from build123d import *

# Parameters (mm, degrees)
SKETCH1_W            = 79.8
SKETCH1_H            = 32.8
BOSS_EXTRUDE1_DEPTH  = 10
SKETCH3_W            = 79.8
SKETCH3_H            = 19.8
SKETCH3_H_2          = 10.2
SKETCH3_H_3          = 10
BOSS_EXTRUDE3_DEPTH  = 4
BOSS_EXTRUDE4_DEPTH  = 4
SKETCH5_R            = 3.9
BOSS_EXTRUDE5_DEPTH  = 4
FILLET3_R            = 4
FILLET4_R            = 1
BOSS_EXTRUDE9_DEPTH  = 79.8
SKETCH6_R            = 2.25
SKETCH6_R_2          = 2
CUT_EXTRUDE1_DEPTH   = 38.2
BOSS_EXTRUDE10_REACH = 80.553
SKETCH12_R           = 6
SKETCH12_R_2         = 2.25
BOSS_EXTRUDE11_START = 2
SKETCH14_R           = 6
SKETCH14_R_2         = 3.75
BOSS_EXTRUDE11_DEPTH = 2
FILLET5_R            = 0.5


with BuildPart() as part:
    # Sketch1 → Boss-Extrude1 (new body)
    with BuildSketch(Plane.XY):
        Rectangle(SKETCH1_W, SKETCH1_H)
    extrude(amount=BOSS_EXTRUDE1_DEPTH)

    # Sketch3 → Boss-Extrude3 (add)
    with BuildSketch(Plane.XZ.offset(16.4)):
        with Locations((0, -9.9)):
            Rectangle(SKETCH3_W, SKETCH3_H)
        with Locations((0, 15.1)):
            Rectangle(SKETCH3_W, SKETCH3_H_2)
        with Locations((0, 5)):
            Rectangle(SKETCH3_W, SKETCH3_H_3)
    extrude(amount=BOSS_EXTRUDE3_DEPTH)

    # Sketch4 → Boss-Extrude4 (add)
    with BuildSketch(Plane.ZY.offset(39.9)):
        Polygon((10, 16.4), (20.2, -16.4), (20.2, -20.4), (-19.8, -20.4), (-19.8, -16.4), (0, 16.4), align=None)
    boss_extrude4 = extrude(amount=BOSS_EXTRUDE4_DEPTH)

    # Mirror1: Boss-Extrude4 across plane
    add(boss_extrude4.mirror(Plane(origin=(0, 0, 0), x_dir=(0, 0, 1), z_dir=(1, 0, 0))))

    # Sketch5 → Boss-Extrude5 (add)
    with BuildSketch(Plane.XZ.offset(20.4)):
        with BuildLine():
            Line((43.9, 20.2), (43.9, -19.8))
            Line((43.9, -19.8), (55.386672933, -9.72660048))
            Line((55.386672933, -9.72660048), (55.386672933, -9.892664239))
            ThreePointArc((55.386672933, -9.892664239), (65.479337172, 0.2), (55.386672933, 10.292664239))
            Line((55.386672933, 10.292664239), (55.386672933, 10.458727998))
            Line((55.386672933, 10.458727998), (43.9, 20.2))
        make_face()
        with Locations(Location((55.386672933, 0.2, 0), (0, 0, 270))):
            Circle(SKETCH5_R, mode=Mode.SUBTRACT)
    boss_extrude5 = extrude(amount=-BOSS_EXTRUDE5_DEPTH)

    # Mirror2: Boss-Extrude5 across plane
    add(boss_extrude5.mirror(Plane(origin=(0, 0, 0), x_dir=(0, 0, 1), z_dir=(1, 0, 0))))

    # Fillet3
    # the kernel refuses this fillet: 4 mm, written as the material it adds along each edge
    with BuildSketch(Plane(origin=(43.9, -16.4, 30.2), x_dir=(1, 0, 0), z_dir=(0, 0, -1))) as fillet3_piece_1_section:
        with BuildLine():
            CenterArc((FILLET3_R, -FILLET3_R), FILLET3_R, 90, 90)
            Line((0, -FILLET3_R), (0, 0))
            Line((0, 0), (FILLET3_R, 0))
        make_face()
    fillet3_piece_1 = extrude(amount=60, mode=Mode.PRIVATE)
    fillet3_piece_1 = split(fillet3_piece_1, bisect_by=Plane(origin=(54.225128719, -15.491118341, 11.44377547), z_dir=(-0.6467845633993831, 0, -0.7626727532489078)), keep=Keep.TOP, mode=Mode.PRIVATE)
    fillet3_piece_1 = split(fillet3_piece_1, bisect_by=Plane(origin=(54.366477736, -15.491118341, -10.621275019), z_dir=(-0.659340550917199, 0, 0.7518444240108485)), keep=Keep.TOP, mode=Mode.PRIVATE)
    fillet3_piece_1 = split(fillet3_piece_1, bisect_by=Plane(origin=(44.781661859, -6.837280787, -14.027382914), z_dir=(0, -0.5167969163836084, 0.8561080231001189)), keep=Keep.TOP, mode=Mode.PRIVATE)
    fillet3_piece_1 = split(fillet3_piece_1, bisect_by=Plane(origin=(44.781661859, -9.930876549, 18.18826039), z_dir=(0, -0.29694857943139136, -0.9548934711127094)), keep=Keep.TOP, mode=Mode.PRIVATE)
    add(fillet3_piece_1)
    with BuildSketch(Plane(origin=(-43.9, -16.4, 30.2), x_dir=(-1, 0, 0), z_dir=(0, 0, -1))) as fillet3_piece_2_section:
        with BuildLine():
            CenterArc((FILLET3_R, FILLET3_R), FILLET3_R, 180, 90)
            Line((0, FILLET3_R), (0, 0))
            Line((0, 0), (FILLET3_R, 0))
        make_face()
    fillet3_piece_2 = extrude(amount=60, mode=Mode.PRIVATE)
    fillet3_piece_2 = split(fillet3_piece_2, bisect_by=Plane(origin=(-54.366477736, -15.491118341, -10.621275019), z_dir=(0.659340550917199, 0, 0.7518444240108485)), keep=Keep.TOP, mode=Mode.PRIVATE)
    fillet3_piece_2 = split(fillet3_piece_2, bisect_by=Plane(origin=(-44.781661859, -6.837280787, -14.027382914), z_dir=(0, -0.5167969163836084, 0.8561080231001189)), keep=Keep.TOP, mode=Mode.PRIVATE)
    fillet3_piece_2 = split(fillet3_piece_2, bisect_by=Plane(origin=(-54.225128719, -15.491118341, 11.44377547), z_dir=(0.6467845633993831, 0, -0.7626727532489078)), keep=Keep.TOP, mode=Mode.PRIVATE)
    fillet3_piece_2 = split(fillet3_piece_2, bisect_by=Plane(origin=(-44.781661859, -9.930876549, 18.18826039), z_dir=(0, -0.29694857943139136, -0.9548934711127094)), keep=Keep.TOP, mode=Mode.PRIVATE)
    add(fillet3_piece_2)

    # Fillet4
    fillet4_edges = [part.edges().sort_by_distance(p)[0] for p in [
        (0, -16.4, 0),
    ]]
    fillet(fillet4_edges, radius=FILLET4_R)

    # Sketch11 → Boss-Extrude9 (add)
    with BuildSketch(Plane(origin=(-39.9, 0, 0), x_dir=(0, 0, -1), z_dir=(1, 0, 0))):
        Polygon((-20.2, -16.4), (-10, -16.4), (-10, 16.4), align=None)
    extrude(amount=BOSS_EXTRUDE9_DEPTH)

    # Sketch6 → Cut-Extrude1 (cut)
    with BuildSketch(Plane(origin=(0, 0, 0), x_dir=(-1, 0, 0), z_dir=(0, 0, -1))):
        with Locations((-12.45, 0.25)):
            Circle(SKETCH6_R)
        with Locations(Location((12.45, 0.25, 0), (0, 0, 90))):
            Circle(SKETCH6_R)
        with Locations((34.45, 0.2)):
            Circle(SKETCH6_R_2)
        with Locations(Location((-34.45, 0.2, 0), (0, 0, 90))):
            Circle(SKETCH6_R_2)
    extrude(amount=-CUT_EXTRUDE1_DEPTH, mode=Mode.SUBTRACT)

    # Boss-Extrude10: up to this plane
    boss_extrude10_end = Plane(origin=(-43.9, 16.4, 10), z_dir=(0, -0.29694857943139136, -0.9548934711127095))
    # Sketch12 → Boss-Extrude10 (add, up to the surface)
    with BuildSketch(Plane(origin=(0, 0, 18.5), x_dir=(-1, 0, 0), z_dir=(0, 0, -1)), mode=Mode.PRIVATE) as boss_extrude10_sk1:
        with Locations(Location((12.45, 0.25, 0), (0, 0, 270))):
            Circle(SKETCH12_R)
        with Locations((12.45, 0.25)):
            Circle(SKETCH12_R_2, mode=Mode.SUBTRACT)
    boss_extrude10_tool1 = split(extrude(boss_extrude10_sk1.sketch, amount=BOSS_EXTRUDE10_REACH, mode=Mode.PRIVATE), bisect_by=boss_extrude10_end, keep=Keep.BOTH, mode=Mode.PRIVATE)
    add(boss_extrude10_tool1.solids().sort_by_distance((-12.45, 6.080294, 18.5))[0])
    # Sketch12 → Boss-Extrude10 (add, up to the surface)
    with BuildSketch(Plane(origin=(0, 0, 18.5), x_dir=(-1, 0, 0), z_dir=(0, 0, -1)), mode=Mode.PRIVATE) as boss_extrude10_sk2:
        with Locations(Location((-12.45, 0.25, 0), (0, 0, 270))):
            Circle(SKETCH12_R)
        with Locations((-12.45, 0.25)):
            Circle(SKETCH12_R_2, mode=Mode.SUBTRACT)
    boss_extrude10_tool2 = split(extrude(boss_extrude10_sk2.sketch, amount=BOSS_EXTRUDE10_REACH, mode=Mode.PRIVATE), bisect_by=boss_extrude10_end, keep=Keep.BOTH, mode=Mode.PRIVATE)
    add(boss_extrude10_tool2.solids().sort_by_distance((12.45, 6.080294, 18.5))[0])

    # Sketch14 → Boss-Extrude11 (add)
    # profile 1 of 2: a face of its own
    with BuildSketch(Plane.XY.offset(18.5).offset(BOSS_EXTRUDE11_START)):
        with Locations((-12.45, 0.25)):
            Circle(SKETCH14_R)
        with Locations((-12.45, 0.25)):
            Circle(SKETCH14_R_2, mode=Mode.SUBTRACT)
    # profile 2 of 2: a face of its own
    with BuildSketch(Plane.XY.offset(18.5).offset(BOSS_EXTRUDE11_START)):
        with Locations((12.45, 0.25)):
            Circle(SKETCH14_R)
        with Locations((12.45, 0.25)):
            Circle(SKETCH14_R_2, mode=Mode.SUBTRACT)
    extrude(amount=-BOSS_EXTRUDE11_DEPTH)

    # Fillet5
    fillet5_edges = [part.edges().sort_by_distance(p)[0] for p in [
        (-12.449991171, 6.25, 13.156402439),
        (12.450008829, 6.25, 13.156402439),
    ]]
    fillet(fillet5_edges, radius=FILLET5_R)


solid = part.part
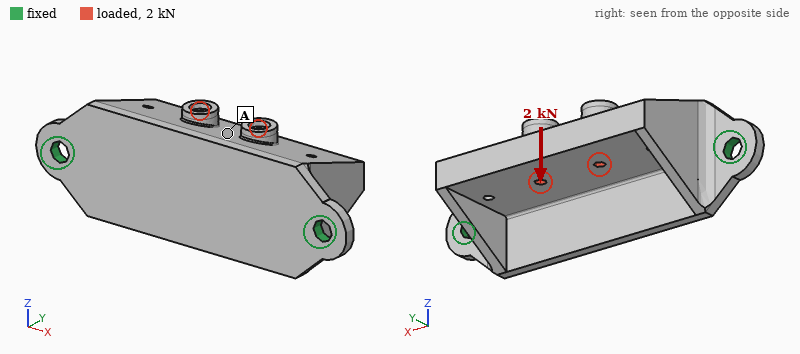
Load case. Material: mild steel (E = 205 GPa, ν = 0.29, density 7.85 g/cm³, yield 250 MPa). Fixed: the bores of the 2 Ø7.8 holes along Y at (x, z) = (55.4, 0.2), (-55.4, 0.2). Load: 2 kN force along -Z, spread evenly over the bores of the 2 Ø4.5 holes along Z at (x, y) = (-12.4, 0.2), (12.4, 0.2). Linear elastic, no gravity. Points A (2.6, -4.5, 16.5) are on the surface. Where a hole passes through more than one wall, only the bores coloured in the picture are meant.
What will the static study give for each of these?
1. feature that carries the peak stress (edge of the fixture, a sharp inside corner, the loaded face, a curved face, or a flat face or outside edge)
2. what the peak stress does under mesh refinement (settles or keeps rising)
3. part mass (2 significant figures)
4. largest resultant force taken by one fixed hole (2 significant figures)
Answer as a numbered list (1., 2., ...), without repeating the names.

1. edge of the fixture
2. keeps rising
3. 500 g
4. 1.0 kN
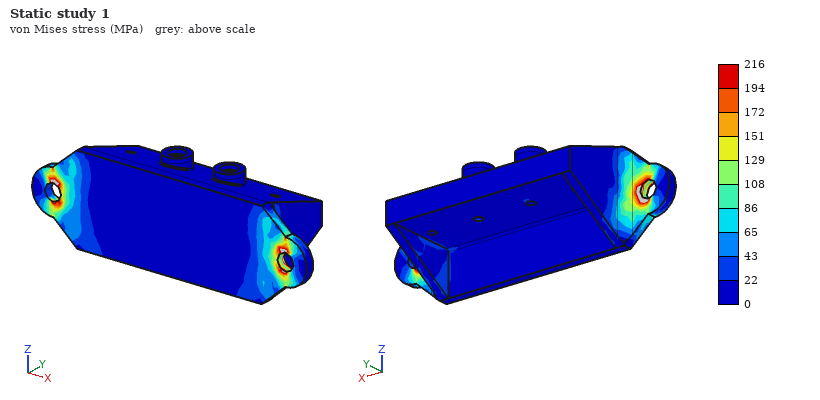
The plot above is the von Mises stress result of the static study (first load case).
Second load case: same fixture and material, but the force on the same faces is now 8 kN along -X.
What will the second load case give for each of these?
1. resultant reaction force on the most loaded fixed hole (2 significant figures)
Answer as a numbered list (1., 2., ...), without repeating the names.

1. 4.3 kN
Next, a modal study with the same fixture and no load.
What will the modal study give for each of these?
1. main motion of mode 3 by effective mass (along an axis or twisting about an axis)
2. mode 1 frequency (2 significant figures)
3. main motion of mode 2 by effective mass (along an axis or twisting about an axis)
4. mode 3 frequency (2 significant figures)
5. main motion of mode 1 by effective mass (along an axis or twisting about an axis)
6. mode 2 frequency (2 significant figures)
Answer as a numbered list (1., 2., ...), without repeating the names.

1. along Z
2. 1400 Hz
3. along Y
4. 6100 Hz
5. along Z
6. 4000 Hz
